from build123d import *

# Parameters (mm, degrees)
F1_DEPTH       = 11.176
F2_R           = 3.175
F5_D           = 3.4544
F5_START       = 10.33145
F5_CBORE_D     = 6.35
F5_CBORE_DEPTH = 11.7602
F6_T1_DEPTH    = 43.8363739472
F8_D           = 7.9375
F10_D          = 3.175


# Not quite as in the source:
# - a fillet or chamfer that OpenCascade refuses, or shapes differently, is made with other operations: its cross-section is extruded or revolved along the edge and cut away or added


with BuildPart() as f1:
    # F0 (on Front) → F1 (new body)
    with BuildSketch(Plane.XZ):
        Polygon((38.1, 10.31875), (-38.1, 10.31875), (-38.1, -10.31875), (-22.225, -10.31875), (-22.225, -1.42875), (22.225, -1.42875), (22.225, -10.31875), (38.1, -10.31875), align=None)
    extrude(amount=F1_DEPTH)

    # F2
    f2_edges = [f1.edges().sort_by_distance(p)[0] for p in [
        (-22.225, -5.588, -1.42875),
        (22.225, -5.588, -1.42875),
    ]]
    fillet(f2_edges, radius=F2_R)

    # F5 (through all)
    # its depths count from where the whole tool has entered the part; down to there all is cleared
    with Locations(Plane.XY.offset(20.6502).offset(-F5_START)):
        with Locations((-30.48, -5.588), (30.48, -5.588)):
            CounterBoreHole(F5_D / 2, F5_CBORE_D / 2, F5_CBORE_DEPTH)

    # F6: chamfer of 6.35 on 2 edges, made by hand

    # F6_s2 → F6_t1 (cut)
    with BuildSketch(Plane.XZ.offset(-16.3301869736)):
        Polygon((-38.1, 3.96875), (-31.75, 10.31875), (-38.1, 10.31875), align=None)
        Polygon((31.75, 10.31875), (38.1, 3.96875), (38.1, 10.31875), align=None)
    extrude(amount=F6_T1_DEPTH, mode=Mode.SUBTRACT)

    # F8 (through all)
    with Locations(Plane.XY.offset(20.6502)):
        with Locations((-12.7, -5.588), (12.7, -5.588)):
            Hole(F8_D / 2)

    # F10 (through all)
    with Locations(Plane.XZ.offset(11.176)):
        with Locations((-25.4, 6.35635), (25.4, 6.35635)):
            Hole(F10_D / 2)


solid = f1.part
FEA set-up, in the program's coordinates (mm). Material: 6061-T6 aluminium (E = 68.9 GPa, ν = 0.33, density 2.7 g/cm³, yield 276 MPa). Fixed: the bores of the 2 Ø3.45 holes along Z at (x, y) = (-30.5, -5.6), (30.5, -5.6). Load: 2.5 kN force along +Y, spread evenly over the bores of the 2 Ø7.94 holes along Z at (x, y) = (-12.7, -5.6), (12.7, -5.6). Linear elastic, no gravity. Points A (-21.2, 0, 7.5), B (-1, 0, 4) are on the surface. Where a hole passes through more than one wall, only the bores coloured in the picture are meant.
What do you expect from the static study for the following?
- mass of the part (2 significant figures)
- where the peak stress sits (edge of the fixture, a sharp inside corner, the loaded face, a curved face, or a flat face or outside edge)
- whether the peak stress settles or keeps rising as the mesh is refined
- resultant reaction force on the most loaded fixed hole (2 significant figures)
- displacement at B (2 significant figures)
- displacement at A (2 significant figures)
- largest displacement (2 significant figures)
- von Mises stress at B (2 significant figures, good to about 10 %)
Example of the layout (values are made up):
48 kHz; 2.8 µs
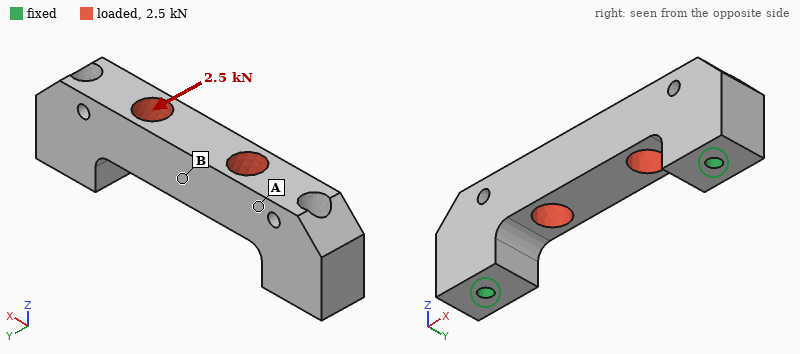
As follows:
28 g; edge of the fixture; keeps rising; 1.3 kN; 78 µm; 40 µm; 88 µm; 42 MPa
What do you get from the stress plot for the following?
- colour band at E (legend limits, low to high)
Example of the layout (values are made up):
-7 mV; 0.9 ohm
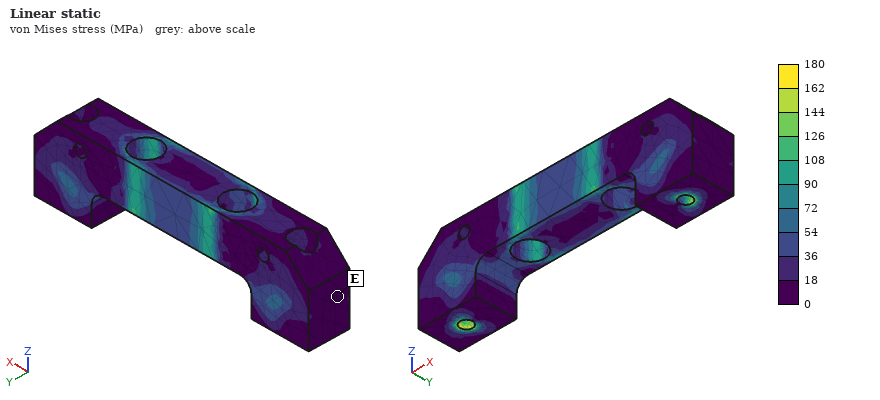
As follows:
0 to 18 MPa
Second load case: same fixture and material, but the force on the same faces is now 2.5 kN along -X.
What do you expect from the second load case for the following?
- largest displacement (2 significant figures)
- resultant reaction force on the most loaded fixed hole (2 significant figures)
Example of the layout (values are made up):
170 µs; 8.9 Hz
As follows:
14 µm; 1.3 kN
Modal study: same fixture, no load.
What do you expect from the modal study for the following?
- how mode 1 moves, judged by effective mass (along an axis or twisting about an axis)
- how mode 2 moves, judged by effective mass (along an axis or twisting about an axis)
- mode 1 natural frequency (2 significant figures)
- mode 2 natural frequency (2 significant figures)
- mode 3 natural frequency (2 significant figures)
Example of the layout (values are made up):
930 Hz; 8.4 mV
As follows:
along Y; along Z; 8100 Hz; 13 kHz; 18 kHz
